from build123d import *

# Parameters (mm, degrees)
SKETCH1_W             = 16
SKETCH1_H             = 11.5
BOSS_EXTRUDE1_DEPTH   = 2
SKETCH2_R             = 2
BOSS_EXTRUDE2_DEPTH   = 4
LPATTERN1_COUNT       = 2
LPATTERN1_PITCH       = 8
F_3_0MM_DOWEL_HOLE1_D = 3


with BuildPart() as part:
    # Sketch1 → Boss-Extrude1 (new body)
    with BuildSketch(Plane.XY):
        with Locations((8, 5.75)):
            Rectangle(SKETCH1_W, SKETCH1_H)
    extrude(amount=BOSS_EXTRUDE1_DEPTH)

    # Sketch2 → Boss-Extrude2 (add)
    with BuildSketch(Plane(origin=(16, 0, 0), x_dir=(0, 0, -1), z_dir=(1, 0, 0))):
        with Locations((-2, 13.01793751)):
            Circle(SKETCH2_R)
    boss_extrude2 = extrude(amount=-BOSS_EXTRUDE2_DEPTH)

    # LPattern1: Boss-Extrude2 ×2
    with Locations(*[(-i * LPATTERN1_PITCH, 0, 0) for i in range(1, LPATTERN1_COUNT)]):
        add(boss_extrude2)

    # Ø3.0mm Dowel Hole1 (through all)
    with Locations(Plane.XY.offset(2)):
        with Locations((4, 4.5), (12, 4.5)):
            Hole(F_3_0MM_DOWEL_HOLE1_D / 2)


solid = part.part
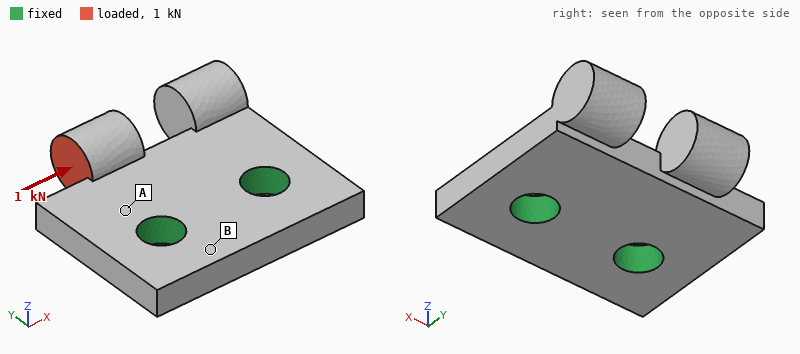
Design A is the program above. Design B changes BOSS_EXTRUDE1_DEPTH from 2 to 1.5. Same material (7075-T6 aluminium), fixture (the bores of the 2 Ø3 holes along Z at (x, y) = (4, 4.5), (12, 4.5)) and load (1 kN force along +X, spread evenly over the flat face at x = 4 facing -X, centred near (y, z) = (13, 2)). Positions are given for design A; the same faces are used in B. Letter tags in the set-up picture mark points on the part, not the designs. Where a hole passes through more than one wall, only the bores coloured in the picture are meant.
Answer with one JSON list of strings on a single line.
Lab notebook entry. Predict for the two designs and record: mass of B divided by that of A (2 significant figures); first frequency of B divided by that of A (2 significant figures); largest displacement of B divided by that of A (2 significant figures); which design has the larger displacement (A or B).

["0.81", "0.67", "1.8", "B"]
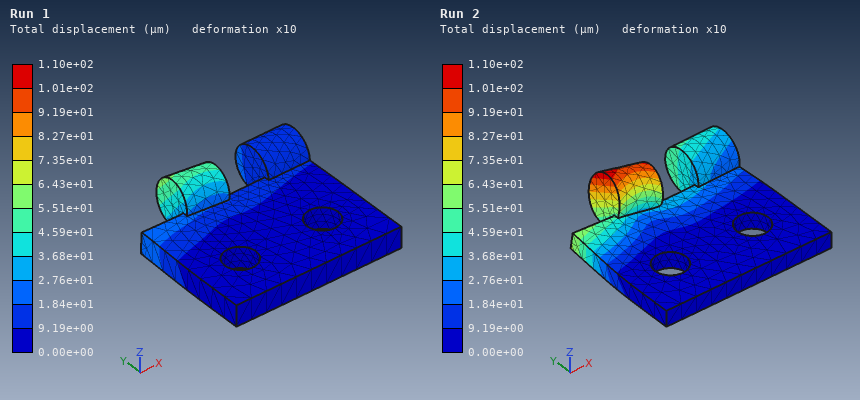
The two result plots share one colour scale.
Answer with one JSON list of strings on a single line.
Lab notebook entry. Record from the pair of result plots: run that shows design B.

["Run 2"]
